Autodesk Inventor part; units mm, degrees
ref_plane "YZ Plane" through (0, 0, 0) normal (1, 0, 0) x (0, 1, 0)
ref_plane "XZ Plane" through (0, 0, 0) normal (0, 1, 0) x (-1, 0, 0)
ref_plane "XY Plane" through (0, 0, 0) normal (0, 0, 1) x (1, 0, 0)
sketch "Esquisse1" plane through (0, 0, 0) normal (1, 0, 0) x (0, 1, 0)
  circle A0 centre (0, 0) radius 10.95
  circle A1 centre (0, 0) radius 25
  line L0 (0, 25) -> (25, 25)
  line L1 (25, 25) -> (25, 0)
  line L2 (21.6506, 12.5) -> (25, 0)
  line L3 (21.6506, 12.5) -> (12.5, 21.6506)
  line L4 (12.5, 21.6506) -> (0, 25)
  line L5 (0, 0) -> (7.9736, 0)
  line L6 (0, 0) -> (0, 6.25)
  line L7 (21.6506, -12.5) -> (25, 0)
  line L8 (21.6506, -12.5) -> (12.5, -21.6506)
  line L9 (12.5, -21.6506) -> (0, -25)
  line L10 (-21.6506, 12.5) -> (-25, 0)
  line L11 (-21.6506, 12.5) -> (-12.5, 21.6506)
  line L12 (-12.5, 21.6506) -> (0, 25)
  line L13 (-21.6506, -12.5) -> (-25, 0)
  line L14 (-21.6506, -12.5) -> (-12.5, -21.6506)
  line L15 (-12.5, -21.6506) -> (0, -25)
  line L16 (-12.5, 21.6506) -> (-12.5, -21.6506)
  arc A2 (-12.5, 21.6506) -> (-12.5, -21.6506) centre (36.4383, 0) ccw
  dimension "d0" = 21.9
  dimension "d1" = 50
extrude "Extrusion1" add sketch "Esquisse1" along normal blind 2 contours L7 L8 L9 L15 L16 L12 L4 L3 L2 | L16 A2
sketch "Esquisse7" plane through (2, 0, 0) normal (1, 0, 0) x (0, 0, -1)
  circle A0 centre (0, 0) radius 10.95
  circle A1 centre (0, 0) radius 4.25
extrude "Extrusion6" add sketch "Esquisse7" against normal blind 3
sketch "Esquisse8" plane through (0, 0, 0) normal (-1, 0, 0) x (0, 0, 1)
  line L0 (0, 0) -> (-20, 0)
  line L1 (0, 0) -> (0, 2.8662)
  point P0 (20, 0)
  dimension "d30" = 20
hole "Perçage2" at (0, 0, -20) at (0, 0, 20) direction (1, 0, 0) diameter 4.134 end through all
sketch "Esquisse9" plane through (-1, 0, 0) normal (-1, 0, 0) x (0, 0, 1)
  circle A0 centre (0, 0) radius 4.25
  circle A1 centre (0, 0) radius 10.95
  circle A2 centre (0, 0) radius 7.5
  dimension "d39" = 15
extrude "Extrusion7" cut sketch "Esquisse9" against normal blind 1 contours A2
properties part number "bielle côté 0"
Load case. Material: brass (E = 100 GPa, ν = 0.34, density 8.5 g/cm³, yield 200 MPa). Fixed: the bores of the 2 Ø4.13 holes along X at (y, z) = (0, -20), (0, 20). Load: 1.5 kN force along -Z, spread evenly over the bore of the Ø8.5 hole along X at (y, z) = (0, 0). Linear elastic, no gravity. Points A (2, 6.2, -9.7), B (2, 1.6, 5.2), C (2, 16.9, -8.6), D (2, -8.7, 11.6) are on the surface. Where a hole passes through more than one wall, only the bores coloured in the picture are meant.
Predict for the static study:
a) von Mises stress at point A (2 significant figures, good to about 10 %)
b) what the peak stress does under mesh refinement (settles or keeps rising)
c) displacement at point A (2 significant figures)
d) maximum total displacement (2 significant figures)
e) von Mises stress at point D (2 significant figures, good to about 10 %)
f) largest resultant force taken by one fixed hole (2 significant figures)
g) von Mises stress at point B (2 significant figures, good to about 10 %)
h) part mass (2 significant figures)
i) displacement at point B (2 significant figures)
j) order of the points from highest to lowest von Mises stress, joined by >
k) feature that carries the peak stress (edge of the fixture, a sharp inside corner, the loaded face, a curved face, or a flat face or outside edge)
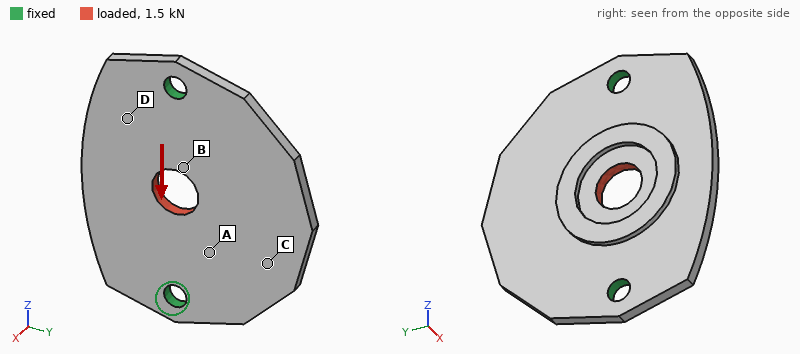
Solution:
17 MPa
keeps rising
3.0 µm
5.2 µm
9.6 MPa
750 N
32 MPa
28 g
4.3 µm
B > A > D > C
edge of the fixture
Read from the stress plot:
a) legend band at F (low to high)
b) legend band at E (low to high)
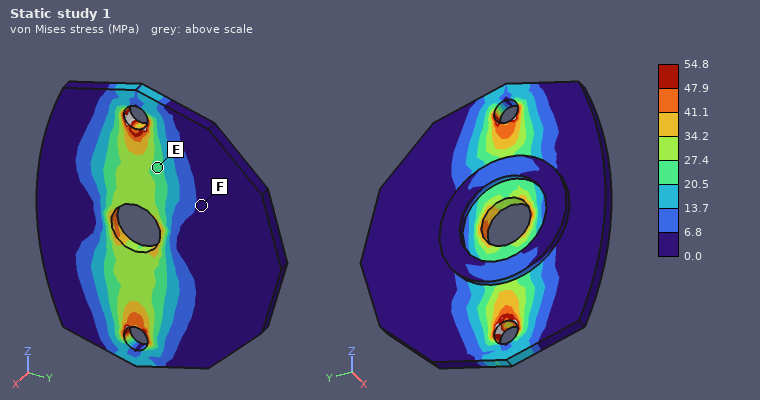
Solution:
0.0 to 6.8 MPa
20.5 to 27.4 MPa
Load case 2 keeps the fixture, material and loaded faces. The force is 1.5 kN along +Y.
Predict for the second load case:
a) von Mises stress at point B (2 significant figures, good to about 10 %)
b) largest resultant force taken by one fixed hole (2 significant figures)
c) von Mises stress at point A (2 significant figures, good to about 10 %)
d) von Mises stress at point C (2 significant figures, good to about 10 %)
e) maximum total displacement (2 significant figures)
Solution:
30 MPa
750 N
20 MPa
15 MPa
9.0 µm
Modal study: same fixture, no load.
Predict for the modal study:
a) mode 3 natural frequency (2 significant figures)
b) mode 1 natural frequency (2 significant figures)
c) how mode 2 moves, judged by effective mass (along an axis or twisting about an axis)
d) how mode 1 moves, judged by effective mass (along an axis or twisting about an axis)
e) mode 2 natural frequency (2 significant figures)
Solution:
5400 Hz
2000 Hz
along X
along X
3400 Hz
